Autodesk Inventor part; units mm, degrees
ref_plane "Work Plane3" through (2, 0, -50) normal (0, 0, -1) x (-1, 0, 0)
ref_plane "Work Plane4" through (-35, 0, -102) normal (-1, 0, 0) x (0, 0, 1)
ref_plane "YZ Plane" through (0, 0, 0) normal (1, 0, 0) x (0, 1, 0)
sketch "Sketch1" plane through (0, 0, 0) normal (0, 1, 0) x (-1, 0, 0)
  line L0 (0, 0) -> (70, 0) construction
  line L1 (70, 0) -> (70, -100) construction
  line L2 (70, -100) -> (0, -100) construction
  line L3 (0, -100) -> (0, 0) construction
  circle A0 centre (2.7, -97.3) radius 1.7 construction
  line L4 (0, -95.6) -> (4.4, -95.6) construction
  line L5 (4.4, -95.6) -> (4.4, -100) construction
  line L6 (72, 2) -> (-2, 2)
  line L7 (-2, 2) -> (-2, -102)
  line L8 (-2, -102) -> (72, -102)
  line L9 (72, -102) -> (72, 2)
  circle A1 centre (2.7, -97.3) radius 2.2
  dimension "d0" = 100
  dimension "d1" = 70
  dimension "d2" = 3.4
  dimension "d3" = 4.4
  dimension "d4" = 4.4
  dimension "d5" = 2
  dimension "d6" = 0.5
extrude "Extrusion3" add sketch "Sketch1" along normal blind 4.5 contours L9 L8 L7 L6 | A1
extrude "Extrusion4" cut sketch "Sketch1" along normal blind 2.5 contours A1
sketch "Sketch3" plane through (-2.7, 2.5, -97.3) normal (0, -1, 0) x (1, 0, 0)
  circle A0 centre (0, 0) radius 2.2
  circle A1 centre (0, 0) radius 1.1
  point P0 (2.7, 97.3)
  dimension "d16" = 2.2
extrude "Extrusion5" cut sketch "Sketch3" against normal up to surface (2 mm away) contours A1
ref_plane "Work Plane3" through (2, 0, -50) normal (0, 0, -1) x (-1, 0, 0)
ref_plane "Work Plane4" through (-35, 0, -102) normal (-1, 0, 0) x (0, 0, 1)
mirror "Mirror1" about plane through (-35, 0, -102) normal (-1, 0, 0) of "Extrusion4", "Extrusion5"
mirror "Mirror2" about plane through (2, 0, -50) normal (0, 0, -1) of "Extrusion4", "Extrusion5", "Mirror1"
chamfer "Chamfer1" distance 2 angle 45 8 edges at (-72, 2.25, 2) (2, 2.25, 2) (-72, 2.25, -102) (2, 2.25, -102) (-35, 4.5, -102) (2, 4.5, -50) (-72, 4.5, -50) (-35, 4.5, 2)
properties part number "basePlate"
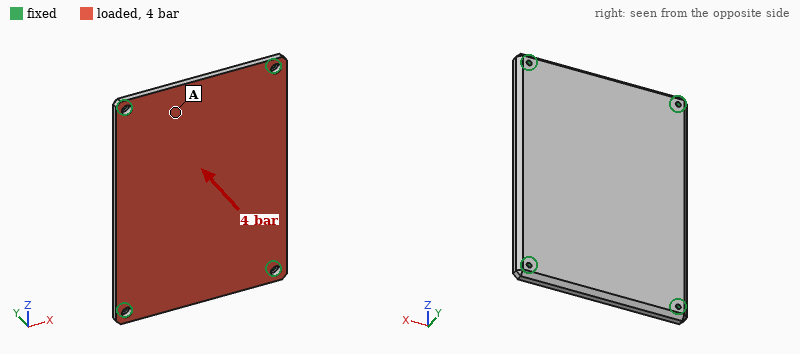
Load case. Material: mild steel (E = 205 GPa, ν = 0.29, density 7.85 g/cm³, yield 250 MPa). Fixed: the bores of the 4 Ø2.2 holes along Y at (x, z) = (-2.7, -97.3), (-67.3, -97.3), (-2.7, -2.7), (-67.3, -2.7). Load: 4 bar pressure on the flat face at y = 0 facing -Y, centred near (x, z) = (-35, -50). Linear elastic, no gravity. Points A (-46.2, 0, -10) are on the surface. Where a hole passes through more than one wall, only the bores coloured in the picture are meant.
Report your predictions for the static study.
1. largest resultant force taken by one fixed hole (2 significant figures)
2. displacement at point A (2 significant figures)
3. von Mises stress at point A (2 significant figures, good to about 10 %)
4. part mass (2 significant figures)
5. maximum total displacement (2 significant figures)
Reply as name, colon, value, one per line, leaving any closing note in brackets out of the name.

largest resultant force taken by one fixed hole: 1.8 kN
displacement at point A: 0.059 mm
von Mises stress at point A: 43 MPa
part mass: 260 g
maximum total displacement: 0.16 mm
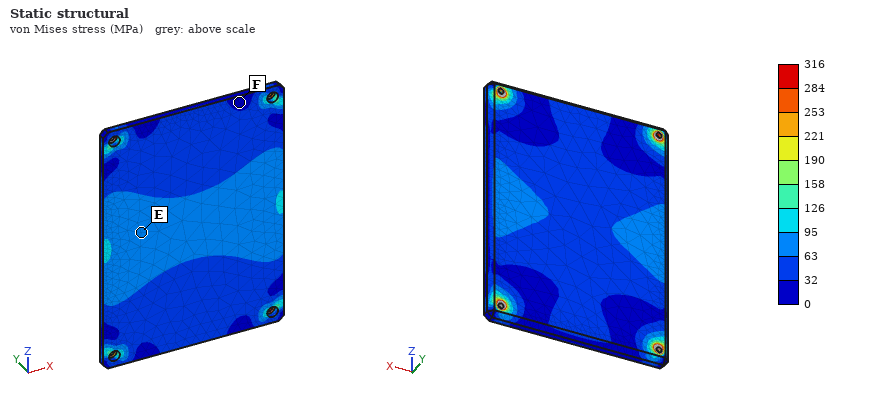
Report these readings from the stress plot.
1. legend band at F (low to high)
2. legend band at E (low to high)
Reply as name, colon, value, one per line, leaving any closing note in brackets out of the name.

legend band at F: 0 to 32 MPa
legend band at E: 63 to 95 MPa
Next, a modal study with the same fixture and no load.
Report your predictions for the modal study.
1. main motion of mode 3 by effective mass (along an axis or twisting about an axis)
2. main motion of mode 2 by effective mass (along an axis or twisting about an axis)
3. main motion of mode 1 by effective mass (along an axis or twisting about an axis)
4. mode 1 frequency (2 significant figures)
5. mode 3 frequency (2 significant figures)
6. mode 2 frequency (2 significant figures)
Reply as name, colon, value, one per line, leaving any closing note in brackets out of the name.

main motion of mode 3 by effective mass: twisting about X
main motion of mode 2 by effective mass: twisting about Z
main motion of mode 1 by effective mass: along Y
mode 1 frequency: 1600 Hz
mode 3 frequency: 3800 Hz
mode 2 frequency: 2800 Hz
